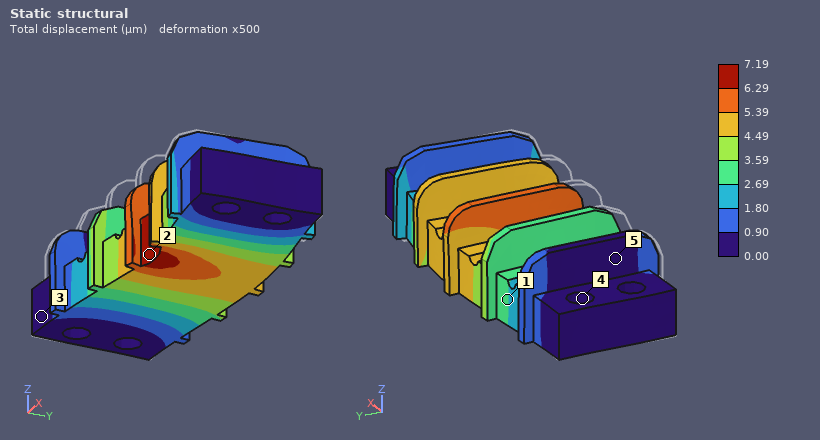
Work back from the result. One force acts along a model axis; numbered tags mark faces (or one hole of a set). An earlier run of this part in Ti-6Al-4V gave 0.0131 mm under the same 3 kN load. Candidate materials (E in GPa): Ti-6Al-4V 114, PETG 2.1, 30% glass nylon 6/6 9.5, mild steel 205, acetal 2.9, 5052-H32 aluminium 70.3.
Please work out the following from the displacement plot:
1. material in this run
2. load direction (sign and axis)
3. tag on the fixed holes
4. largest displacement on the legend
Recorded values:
mild steel
+Y
4
7.19 µm
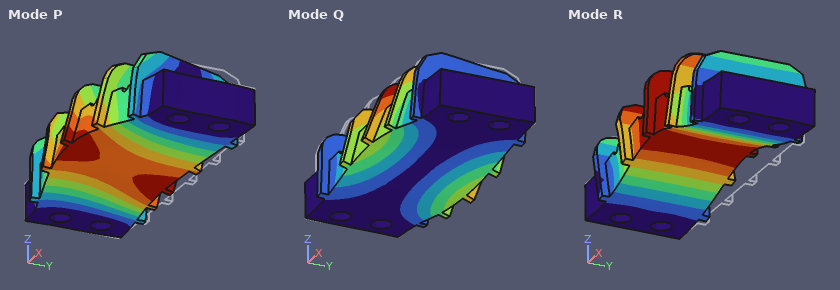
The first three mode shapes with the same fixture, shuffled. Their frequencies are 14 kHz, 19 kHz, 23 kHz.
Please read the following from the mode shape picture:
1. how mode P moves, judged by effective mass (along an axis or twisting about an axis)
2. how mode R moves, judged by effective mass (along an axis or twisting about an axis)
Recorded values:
along Y
along Z
